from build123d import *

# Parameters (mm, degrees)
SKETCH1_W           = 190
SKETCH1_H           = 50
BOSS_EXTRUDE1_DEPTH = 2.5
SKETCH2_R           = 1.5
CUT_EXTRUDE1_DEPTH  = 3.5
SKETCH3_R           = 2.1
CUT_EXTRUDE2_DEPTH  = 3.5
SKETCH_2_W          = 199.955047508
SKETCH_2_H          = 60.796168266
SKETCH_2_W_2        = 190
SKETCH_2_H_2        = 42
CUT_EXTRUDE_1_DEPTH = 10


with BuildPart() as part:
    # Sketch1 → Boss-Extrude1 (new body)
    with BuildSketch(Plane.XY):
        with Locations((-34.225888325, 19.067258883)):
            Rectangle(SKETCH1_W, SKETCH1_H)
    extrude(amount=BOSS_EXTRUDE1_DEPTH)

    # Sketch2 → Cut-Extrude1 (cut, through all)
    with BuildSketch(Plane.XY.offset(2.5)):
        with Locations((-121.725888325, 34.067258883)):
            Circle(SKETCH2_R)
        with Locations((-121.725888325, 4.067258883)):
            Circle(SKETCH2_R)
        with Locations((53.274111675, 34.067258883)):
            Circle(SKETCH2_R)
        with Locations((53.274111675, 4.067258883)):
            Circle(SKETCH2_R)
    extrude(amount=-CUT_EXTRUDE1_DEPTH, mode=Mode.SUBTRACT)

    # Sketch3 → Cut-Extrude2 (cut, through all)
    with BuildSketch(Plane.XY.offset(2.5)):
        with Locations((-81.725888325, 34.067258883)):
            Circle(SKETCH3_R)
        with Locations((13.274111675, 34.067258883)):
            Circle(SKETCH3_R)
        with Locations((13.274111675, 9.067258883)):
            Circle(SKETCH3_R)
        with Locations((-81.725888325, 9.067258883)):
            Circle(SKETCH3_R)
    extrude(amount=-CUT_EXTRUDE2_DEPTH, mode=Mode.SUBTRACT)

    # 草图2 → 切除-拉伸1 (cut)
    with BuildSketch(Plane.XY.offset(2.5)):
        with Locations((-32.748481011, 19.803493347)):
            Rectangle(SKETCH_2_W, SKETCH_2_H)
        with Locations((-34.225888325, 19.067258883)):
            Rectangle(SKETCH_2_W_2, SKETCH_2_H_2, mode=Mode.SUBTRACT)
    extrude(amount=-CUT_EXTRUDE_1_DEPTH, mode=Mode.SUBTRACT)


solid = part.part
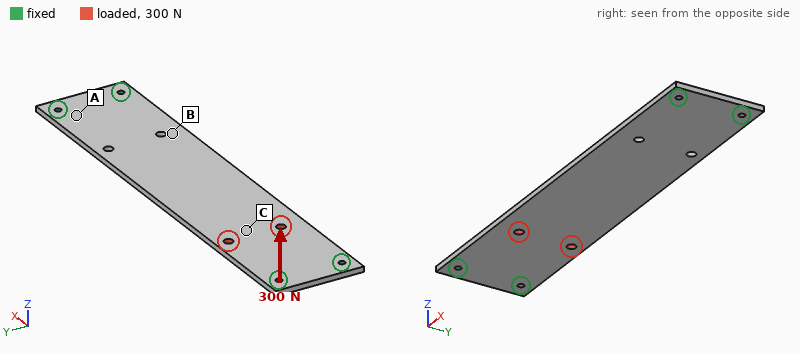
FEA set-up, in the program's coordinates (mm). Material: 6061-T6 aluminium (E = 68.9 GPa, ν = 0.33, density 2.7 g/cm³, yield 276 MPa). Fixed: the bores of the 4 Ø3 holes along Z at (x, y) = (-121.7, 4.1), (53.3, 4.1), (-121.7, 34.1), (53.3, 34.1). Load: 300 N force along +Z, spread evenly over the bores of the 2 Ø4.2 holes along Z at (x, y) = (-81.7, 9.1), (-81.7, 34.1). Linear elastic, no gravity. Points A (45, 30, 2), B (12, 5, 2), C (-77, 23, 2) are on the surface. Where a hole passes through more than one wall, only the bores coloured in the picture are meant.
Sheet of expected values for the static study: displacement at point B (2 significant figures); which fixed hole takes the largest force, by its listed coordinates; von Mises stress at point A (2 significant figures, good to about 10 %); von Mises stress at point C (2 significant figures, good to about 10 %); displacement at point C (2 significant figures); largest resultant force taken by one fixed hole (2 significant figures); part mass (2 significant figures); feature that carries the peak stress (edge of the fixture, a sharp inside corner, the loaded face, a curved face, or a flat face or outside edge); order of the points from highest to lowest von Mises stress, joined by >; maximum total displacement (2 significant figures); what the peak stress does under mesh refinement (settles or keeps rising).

0.37 mm
(-121.7, 34.1)
39 MPa
72 MPa
0.91 mm
150 N
53 g
edge of the fixture
C > A > B
1.2 mm
keeps rising
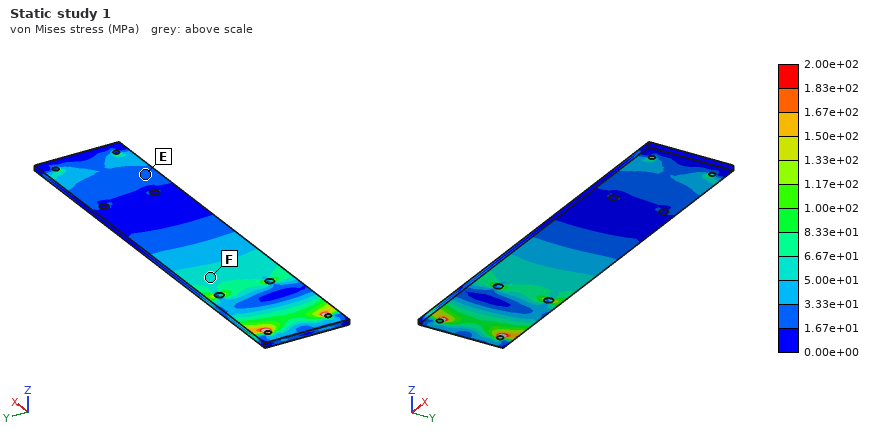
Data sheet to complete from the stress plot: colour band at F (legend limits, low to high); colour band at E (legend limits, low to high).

5.00e+01 to 6.67e+01 MPa
1.67e+01 to 3.33e+01 MPa
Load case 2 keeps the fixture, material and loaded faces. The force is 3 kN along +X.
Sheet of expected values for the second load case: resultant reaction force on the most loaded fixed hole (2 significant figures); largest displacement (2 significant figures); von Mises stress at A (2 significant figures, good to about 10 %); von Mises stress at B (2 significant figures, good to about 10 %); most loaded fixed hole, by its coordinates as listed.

1.2 kN
20 µm
7.8 MPa
8.4 MPa
(-121.7, 34.1)
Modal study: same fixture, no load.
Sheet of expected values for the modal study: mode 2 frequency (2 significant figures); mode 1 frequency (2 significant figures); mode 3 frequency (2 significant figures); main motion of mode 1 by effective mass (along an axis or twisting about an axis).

1200 Hz
420 Hz
1200 Hz
along Z
